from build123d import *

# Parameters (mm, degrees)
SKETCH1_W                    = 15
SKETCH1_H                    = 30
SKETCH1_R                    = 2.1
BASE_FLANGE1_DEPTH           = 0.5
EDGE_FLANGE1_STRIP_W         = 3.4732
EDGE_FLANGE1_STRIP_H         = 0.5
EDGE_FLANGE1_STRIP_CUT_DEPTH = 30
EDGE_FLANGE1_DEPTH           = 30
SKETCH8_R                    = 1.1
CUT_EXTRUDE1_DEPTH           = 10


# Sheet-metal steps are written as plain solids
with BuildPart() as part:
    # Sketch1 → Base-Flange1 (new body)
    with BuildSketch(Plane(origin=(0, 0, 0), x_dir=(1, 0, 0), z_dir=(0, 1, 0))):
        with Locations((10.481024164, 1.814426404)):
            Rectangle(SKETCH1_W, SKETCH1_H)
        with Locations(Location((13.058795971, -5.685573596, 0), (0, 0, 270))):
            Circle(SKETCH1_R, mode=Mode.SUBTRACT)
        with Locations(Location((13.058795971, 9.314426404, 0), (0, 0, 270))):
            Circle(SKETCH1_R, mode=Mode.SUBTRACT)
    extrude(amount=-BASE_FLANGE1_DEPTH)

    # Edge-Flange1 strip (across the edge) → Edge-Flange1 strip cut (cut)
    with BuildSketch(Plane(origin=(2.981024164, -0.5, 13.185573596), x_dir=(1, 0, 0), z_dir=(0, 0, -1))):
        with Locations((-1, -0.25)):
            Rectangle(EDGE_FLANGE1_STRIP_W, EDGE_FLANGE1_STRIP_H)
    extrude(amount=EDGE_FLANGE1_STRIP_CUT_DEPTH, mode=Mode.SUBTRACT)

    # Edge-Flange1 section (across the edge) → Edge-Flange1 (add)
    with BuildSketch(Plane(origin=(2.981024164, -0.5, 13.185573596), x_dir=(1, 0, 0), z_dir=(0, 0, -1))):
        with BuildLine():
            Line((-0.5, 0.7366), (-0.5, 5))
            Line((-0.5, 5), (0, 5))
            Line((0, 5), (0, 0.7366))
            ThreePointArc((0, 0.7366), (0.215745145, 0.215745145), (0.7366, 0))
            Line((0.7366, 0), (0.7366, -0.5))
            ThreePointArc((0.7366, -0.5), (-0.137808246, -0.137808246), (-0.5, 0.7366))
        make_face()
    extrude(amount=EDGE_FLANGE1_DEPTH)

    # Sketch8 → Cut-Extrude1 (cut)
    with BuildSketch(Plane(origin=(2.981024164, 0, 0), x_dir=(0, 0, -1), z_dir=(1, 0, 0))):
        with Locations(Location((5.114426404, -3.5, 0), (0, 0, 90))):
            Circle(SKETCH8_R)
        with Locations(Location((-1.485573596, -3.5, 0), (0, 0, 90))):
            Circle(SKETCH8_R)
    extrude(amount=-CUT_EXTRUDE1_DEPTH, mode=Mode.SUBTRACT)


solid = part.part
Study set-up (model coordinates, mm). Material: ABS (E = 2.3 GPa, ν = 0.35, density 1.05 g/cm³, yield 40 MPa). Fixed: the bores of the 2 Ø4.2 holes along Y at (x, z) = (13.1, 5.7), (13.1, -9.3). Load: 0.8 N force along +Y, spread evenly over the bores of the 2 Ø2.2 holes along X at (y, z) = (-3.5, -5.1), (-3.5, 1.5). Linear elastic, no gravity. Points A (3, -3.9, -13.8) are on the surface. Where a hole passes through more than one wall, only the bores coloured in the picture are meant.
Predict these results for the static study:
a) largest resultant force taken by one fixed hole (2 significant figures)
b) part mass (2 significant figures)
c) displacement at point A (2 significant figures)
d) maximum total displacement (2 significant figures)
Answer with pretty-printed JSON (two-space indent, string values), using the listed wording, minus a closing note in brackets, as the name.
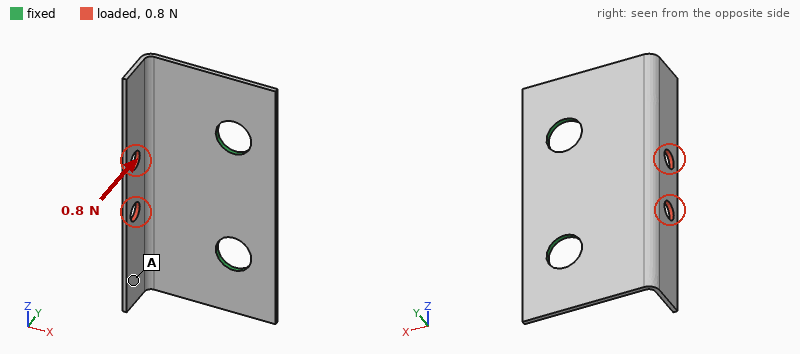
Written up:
{
  "largest resultant force taken by one fixed hole": "0.40 N",
  "part mass": "0.30 g",
  "displacement at point A": "0.29 mm",
  "maximum total displacement": "0.35 mm"
}
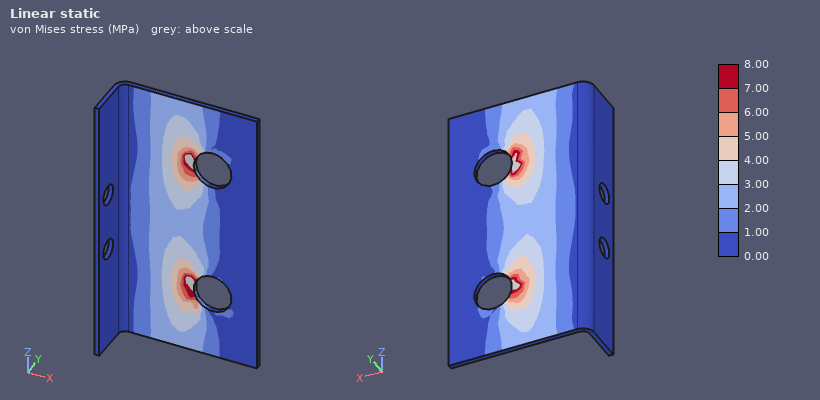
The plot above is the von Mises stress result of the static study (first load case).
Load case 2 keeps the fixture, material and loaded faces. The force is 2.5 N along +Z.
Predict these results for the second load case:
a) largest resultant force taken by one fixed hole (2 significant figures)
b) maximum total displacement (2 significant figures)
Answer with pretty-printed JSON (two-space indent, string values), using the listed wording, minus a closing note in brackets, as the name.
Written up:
{
  "largest resultant force taken by one fixed hole": "1.8 N",
  "maximum total displacement": "0.37 mm"
}
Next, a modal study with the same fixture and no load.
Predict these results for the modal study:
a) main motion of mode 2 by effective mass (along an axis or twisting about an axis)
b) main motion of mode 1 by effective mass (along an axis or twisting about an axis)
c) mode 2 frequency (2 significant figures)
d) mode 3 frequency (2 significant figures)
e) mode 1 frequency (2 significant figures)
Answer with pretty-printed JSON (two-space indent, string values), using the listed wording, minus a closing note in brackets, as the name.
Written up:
{
  "main motion of mode 2 by effective mass": "twisting about X",
  "main motion of mode 1 by effective mass": "along Y",
  "mode 2 frequency": "980 Hz",
  "mode 3 frequency": "2800 Hz",
  "mode 1 frequency": "780 Hz"
}
